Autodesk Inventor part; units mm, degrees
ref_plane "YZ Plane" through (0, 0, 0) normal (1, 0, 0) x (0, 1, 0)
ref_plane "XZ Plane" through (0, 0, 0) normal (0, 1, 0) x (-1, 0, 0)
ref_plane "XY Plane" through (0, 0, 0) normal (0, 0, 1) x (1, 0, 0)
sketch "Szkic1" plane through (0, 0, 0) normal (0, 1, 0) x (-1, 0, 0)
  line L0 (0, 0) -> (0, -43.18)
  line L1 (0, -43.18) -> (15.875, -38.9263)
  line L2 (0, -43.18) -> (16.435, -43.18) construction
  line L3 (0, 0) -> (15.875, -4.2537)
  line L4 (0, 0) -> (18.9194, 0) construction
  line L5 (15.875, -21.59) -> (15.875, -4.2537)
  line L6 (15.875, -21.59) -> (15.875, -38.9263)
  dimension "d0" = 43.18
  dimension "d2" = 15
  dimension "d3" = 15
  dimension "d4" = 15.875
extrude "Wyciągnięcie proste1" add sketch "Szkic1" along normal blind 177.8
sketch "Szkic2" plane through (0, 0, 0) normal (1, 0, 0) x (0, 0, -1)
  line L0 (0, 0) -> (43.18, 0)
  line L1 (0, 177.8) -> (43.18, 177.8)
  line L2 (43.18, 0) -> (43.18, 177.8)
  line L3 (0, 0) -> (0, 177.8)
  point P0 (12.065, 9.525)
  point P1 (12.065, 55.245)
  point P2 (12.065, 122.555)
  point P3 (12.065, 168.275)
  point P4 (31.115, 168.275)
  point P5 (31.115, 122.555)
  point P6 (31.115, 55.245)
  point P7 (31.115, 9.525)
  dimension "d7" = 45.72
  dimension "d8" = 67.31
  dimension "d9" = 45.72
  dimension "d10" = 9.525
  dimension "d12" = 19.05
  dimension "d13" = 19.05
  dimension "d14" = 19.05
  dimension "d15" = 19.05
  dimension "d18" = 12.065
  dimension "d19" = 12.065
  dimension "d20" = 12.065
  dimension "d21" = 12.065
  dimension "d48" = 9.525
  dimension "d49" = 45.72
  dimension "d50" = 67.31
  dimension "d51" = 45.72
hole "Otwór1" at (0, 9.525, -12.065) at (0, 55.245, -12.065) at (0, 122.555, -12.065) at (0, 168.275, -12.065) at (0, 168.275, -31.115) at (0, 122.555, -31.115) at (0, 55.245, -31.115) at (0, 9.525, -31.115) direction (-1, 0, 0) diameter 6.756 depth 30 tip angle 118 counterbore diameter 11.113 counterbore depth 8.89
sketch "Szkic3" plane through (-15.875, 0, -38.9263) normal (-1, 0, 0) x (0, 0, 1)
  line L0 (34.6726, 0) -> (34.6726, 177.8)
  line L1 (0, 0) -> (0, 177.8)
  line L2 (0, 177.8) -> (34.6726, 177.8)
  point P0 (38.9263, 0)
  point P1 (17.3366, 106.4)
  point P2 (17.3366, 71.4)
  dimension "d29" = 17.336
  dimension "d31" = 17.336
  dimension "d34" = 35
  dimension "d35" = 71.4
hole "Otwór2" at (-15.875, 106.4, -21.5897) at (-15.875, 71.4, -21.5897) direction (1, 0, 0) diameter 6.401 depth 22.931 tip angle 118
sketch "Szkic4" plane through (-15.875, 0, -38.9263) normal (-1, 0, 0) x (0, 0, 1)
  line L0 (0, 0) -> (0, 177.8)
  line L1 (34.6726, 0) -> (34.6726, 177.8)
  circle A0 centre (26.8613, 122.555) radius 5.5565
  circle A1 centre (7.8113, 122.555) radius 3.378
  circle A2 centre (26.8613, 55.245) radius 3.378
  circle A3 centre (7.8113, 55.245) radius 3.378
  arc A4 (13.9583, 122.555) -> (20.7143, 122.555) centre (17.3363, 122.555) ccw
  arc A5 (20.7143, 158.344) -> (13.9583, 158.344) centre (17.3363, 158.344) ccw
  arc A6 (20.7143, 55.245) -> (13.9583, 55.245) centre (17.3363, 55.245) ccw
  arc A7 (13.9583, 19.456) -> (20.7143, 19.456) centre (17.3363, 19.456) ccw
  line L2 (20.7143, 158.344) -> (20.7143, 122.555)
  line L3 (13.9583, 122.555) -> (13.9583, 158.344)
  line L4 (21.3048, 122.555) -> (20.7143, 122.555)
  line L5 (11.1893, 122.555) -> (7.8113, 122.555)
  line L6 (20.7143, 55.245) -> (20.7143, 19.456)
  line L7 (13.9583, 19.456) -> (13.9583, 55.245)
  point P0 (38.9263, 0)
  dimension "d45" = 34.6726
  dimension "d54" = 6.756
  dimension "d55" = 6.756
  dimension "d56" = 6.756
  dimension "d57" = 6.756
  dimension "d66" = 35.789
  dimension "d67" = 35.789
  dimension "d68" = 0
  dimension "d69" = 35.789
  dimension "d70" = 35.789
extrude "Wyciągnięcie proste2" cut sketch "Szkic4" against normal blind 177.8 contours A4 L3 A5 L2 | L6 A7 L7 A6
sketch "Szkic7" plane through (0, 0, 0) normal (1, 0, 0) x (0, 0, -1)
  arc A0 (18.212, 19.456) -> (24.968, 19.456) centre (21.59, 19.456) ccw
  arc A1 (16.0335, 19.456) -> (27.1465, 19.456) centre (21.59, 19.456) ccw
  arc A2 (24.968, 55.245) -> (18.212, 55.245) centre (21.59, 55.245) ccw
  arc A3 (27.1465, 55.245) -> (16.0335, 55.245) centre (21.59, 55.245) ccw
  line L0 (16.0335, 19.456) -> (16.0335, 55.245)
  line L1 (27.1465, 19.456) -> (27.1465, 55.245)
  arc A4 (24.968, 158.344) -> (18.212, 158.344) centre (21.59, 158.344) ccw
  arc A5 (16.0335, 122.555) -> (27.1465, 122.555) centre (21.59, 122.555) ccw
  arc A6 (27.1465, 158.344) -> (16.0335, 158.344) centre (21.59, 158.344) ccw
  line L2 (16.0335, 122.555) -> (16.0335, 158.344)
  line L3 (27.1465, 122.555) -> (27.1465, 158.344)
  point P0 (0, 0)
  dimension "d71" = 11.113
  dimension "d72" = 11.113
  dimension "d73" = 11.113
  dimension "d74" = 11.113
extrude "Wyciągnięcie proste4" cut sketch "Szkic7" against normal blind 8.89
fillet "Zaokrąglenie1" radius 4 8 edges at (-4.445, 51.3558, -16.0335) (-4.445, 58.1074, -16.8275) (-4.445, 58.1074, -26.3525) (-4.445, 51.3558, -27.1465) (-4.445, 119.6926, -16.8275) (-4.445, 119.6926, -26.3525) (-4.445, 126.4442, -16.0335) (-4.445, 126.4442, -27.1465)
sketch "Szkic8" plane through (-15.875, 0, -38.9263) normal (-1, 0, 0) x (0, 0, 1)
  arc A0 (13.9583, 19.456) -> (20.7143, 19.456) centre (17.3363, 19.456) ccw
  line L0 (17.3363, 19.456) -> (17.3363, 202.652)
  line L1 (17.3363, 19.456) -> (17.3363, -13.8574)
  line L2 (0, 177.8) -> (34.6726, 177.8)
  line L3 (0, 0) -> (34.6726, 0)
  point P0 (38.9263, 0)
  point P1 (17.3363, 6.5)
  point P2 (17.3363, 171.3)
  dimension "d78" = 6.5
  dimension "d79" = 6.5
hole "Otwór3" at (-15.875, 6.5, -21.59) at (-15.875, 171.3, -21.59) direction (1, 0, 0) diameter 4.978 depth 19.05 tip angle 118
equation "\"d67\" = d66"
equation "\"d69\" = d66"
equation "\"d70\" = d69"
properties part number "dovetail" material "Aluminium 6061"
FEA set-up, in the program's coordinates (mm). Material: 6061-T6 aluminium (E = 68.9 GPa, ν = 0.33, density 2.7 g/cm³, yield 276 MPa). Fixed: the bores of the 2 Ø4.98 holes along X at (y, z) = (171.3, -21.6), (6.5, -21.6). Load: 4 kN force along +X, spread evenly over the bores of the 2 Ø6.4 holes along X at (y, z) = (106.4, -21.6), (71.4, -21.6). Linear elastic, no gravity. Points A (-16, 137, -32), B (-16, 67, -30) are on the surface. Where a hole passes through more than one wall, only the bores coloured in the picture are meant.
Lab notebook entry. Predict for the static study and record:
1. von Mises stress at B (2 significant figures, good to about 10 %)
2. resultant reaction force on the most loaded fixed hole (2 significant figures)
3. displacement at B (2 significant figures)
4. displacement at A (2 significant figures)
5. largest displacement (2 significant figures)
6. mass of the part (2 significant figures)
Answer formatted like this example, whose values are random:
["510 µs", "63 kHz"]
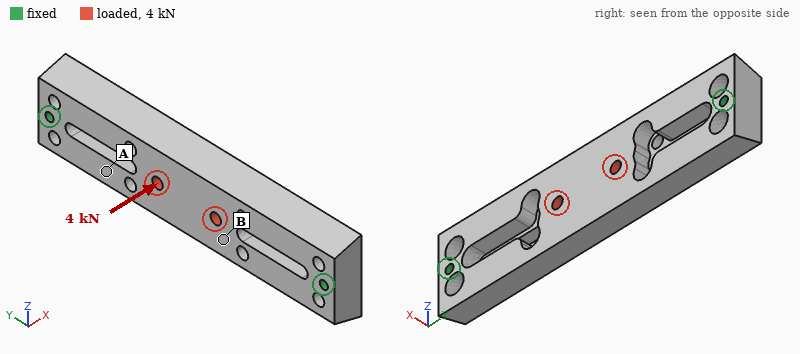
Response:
["35 MPa", "2.1 kN", "0.18 mm", "0.10 mm", "0.20 mm", "230 g"]
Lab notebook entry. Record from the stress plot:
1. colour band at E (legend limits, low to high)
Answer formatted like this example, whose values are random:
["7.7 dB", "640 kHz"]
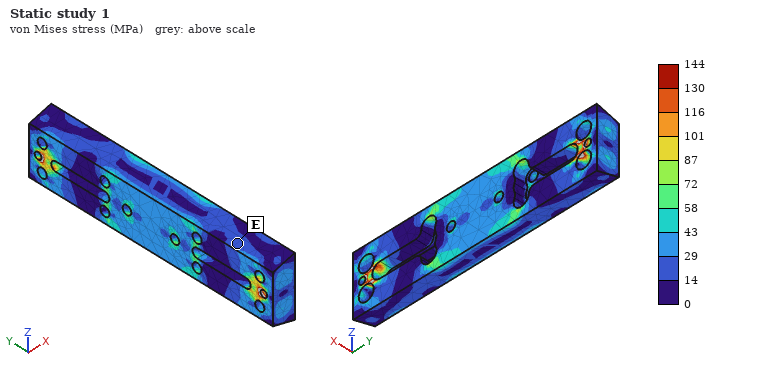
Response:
["14 to 29 MPa"]
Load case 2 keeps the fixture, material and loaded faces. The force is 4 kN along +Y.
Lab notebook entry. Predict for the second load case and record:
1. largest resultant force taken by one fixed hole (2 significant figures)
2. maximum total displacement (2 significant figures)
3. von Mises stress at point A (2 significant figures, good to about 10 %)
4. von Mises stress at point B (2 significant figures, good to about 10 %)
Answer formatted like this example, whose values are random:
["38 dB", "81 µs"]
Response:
["2.0 kN", "11 µm", "5.6 MPa", "3.1 MPa"]
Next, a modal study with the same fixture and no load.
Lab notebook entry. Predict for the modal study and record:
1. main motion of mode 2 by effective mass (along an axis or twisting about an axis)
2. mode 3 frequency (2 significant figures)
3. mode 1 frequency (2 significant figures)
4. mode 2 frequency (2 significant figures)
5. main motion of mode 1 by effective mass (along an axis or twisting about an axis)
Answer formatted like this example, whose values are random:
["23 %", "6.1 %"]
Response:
["along Z", "3800 Hz", "2100 Hz", "2700 Hz", "along X"]
